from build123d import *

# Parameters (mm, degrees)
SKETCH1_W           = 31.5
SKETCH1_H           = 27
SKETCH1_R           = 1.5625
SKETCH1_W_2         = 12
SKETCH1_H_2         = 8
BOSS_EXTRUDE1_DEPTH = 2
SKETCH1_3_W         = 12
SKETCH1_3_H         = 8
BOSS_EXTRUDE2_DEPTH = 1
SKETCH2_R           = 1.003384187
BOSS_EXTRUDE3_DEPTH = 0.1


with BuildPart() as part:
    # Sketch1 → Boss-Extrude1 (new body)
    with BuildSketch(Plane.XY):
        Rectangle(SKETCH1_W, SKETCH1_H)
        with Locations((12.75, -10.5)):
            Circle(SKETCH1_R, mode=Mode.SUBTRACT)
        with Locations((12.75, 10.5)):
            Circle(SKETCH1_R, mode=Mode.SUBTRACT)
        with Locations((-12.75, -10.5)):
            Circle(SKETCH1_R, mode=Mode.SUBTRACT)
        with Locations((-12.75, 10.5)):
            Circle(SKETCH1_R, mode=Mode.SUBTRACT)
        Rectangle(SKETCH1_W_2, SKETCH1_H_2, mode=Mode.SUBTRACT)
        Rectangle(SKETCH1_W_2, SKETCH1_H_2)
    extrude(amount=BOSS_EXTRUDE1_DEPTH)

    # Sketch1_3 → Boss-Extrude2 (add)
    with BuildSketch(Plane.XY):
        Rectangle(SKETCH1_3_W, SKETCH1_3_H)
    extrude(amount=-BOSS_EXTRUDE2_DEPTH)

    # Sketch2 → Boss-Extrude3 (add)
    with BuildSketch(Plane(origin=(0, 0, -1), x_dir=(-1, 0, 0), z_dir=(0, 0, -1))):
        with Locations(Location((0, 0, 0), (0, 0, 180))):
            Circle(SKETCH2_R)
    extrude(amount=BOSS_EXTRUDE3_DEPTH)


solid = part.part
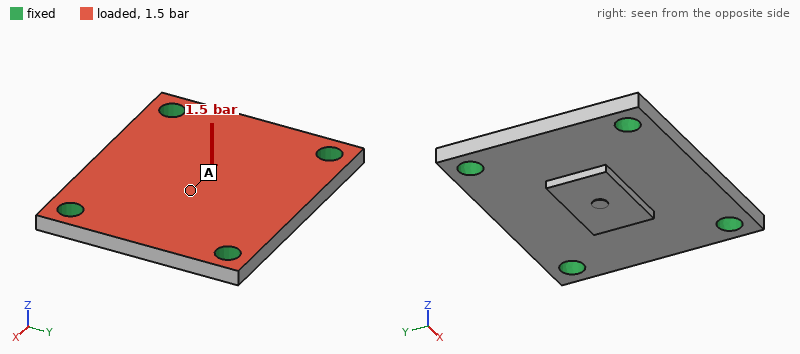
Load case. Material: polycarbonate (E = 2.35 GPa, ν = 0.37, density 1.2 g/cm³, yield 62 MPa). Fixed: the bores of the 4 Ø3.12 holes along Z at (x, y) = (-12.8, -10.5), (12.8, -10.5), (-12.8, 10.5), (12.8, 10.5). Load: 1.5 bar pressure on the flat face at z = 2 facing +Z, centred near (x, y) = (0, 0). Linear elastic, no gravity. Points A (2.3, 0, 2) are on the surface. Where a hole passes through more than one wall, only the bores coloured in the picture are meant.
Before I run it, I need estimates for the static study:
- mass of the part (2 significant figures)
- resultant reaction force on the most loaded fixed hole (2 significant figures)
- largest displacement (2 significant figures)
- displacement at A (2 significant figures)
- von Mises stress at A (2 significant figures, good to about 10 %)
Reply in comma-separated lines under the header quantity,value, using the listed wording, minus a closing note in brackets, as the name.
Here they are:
quantity,value
mass of the part,2.1 g
resultant reaction force on the most loaded fixed hole,31 N
largest displacement,0.11 mm
displacement at A,0.11 mm
von Mises stress at A,3.0 MPa
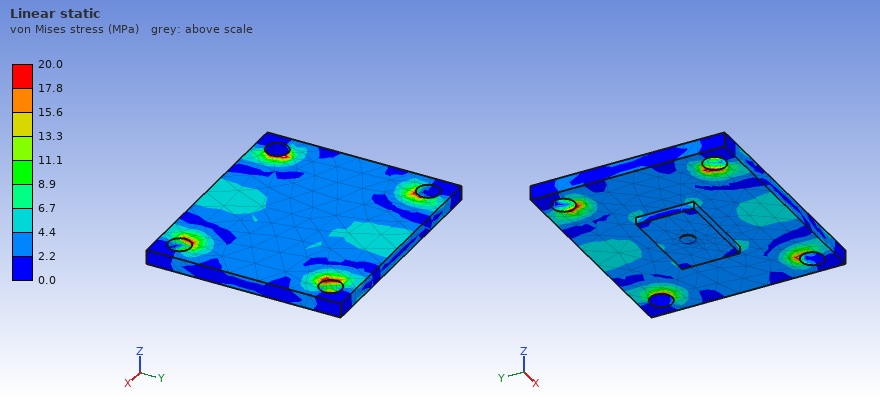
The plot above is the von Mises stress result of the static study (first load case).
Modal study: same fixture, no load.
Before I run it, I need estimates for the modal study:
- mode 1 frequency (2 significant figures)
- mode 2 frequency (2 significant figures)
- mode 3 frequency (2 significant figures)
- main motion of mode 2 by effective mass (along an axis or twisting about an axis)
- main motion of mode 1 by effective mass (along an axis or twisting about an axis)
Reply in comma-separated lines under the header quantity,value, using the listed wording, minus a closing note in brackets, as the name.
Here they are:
quantity,value
mode 1 frequency,4000 Hz
mode 2 frequency,5800 Hz
mode 3 frequency,7400 Hz
main motion of mode 2 by effective mass,twisting about X
main motion of mode 1 by effective mass,along Z
